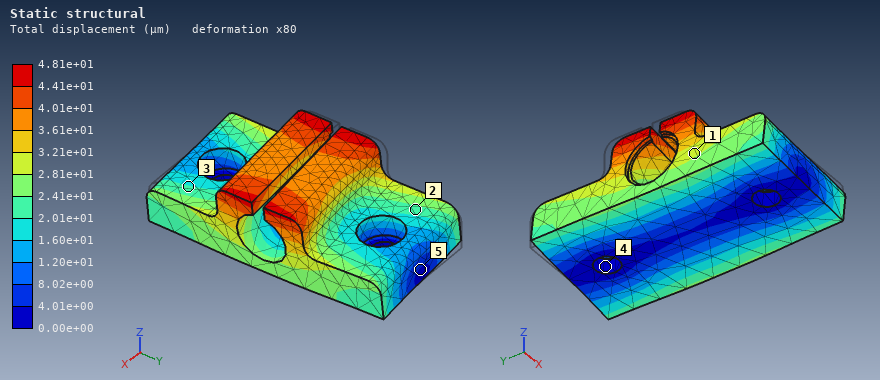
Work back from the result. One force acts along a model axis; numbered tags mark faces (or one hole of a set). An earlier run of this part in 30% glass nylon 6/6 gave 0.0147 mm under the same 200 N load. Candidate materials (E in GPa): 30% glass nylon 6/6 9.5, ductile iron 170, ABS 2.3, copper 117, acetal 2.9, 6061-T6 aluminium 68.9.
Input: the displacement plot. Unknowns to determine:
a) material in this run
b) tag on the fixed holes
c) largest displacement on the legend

acetal
4
4.81e+01 µm
